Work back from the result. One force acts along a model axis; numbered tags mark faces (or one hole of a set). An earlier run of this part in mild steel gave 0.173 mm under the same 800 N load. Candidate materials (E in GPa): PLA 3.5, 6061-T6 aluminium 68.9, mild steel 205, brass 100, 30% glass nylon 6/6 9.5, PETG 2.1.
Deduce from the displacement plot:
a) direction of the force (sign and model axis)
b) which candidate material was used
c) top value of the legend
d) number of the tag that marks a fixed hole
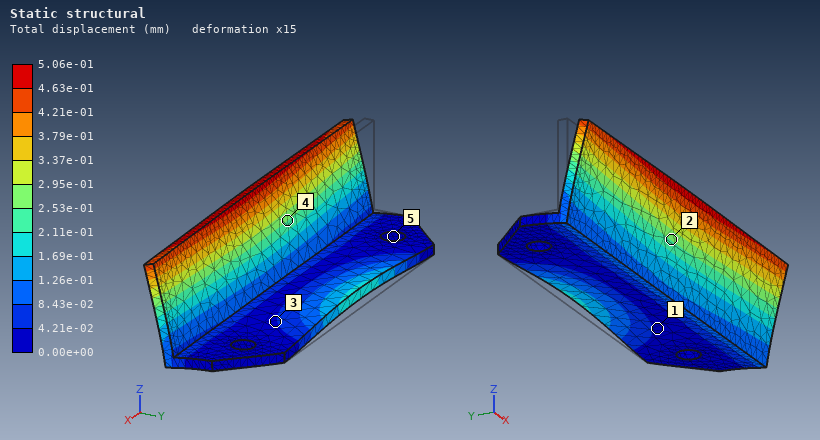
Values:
-Y
6061-T6 aluminium
5.06e-01 mm
5
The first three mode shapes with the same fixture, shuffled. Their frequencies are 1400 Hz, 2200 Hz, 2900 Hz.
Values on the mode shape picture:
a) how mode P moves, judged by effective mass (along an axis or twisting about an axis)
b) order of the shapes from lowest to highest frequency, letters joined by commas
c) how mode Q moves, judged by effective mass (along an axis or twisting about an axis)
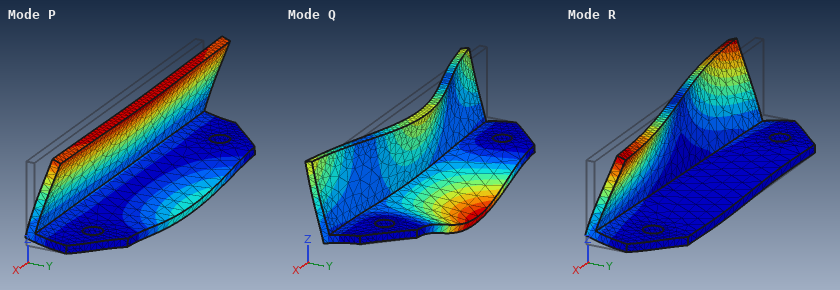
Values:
along Y
P, R, Q
along Z
